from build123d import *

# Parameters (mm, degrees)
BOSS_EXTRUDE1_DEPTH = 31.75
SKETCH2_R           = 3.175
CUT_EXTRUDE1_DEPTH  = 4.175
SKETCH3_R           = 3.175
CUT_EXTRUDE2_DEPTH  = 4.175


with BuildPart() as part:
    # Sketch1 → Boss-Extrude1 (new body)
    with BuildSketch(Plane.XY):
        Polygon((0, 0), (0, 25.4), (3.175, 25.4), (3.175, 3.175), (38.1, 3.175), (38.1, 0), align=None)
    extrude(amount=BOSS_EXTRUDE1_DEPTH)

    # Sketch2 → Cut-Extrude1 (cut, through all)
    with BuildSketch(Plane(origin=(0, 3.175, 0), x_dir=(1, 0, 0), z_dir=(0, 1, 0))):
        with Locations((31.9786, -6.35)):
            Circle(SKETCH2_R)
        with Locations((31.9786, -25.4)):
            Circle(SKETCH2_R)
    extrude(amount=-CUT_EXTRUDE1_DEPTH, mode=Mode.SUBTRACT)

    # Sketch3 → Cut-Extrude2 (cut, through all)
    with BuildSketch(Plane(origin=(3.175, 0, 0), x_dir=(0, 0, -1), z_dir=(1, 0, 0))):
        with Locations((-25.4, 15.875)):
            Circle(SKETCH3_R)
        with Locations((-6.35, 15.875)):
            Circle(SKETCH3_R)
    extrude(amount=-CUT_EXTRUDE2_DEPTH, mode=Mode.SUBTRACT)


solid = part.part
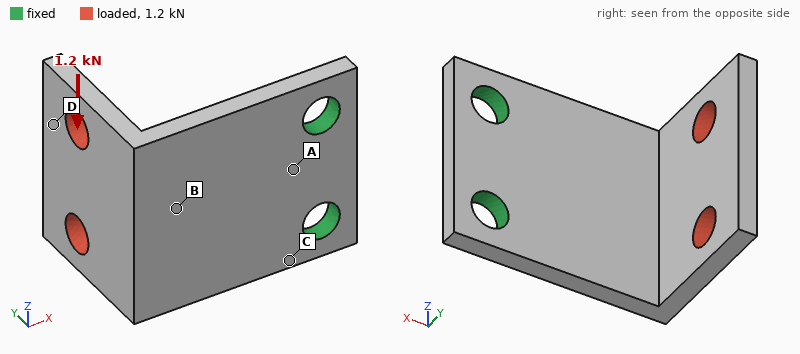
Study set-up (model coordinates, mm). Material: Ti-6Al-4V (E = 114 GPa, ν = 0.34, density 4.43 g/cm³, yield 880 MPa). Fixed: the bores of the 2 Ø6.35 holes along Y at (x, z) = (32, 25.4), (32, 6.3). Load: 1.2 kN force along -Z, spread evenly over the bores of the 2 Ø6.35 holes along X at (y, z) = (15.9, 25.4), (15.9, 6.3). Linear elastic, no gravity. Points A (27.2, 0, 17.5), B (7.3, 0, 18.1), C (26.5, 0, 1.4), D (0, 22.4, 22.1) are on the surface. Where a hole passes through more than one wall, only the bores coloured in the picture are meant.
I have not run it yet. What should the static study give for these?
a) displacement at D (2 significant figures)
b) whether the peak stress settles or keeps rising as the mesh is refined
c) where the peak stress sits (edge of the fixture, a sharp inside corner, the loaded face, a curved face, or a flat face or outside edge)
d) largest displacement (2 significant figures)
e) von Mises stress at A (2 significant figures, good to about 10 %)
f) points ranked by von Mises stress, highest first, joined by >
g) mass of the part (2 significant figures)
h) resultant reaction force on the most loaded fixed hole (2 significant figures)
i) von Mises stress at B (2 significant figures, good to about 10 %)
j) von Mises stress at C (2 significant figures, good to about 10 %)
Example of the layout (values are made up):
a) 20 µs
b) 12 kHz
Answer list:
a) 0.48 mm
b) keeps rising
c) edge of the fixture
d) 0.64 mm
e) 64 MPa
f) C > B > A > D
g) 25 g
h) 1.8 kN
i) 170 MPa
j) 270 MPa
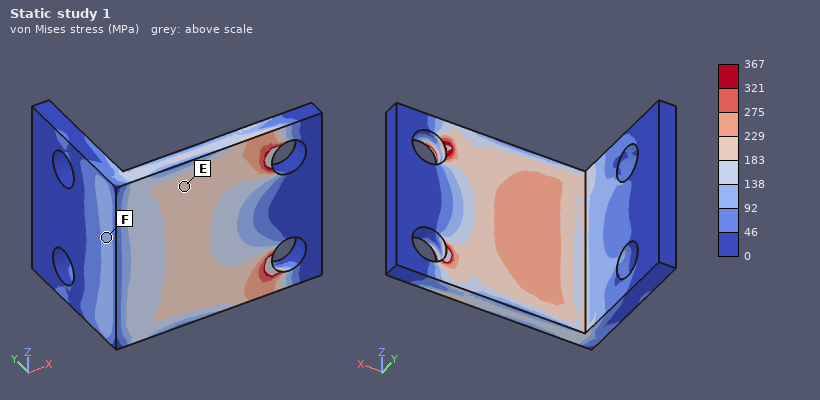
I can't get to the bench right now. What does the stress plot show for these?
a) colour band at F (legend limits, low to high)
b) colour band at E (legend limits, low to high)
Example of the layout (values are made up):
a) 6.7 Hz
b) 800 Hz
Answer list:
a) 92 to 138 MPa
b) 183 to 229 MPa
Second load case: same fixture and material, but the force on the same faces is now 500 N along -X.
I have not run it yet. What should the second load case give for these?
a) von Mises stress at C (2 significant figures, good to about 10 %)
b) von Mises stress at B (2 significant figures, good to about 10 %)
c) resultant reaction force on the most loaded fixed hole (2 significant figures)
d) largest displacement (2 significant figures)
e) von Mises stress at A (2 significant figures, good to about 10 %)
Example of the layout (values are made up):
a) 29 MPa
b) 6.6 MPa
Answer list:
a) 110 MPa
b) 120 MPa
c) 250 N
d) 0.64 mm
e) 95 MPa
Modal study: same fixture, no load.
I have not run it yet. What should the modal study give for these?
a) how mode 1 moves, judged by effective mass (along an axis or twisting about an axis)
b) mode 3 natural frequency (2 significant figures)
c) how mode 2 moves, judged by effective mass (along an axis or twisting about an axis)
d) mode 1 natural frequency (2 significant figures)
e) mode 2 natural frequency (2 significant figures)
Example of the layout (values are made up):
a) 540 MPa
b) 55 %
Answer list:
a) along Y
b) 3900 Hz
c) along Z
d) 1300 Hz
e) 2600 Hz
